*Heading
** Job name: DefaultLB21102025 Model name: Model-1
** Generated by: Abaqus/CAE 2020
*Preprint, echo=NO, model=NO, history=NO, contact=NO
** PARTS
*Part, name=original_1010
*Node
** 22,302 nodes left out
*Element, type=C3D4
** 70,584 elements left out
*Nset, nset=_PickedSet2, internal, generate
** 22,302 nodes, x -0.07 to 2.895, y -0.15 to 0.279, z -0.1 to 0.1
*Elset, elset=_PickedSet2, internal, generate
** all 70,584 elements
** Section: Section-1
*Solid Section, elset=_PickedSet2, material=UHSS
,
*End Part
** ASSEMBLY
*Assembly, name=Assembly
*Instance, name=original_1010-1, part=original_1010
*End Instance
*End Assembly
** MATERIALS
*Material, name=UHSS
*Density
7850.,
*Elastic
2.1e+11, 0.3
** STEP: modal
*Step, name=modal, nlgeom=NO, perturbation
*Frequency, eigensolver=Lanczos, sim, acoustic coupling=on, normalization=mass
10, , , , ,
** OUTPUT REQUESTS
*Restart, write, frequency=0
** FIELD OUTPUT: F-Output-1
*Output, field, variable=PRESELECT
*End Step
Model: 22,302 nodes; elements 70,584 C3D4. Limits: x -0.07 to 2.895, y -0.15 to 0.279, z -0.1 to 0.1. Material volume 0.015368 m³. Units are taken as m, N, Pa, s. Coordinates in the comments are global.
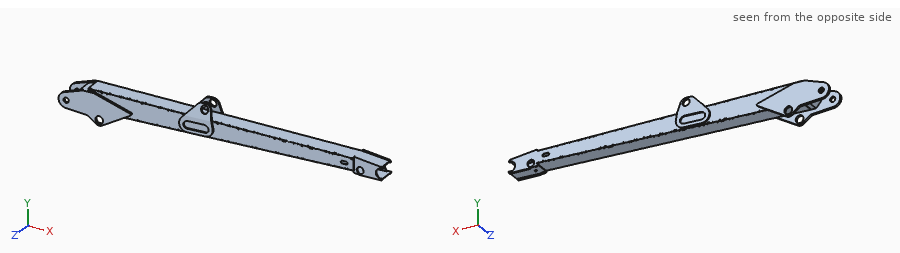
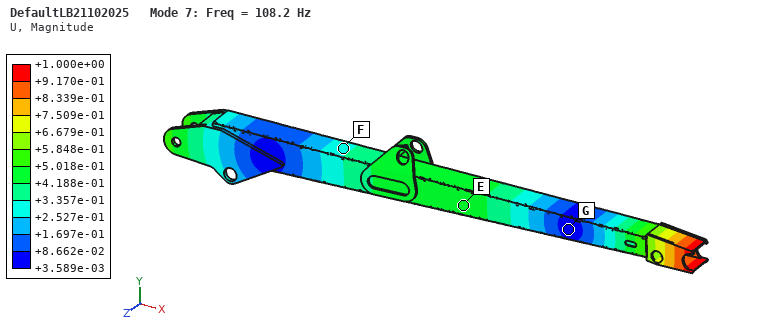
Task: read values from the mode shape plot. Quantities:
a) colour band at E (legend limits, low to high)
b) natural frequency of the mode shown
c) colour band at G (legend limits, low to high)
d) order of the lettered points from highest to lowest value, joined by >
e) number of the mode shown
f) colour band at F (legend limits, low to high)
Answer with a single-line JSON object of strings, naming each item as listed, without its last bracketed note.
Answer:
{"colour band at E": "+4.188e-01 to +5.018e-01", "natural frequency of the mode shown": "108.2 Hz", "colour band at G": "+3.589e-03 to +8.662e-02", "order of the lettered points from highest to lowest value, joined by >": "E > F > G", "number of the mode shown": "7", "colour band at F": "+2.527e-01 to +3.357e-01"}
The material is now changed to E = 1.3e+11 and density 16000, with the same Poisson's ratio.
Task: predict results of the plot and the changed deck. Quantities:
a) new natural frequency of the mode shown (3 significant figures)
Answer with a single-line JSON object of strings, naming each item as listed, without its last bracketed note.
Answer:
{"new natural frequency of the mode shown": "59.6 Hz"}
